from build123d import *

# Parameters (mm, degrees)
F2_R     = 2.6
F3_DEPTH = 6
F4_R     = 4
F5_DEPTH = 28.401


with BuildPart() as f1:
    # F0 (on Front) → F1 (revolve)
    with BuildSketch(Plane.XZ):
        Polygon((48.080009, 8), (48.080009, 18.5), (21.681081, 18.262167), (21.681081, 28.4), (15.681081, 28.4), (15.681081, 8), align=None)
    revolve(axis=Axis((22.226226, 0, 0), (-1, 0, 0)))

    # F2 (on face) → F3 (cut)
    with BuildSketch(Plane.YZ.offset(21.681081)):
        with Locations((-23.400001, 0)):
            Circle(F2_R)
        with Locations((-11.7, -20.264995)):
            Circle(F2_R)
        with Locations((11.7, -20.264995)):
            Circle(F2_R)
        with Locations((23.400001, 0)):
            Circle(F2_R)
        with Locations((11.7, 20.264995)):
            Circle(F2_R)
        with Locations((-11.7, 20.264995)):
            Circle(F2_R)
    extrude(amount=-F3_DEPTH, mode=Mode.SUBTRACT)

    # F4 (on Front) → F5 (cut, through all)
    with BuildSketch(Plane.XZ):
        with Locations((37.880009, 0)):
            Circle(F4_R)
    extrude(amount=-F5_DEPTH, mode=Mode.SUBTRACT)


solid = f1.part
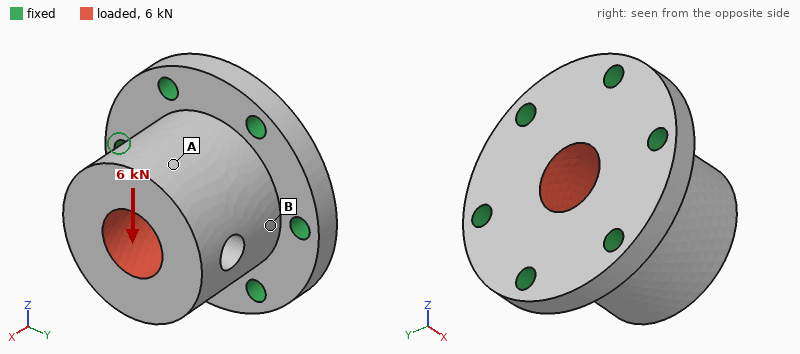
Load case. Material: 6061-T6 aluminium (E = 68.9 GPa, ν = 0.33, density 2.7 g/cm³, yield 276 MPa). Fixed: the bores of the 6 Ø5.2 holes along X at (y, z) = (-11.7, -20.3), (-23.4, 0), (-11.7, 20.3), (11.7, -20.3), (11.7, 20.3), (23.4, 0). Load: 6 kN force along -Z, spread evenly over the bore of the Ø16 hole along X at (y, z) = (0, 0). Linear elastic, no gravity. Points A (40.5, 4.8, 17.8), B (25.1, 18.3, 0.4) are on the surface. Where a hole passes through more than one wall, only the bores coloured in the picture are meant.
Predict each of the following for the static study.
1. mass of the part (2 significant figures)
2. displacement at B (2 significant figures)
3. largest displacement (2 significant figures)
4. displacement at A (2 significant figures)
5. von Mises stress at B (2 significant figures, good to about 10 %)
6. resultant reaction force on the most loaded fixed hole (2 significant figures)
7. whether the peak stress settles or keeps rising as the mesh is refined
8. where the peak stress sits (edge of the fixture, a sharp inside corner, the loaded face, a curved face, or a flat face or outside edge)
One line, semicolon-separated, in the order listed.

96 g; 3.6 µm; 17 µm; 13 µm; 11 MPa; 1.7 kN; keeps rising; edge of the fixture
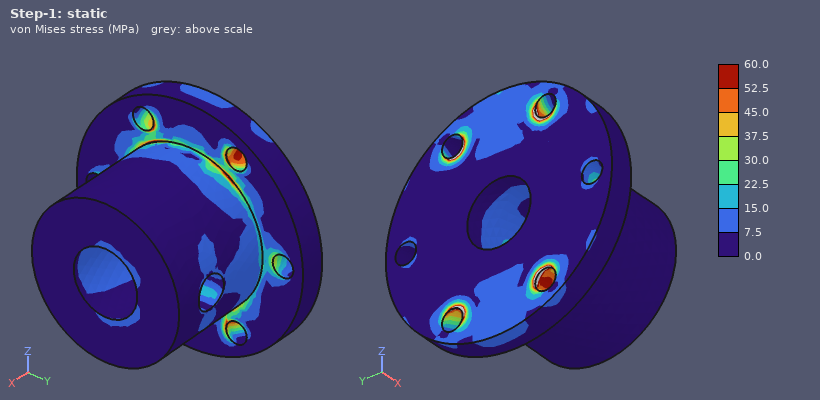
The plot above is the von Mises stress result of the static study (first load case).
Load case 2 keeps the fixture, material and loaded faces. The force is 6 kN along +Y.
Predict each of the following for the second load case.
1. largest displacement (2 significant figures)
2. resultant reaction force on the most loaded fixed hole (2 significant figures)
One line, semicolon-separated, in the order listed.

16 µm; 1.9 kN
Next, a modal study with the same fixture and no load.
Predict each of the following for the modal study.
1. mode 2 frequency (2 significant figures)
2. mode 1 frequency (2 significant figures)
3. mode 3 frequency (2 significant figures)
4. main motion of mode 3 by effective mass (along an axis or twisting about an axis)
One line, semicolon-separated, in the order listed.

13 kHz; 13 kHz; 19 kHz; along X
